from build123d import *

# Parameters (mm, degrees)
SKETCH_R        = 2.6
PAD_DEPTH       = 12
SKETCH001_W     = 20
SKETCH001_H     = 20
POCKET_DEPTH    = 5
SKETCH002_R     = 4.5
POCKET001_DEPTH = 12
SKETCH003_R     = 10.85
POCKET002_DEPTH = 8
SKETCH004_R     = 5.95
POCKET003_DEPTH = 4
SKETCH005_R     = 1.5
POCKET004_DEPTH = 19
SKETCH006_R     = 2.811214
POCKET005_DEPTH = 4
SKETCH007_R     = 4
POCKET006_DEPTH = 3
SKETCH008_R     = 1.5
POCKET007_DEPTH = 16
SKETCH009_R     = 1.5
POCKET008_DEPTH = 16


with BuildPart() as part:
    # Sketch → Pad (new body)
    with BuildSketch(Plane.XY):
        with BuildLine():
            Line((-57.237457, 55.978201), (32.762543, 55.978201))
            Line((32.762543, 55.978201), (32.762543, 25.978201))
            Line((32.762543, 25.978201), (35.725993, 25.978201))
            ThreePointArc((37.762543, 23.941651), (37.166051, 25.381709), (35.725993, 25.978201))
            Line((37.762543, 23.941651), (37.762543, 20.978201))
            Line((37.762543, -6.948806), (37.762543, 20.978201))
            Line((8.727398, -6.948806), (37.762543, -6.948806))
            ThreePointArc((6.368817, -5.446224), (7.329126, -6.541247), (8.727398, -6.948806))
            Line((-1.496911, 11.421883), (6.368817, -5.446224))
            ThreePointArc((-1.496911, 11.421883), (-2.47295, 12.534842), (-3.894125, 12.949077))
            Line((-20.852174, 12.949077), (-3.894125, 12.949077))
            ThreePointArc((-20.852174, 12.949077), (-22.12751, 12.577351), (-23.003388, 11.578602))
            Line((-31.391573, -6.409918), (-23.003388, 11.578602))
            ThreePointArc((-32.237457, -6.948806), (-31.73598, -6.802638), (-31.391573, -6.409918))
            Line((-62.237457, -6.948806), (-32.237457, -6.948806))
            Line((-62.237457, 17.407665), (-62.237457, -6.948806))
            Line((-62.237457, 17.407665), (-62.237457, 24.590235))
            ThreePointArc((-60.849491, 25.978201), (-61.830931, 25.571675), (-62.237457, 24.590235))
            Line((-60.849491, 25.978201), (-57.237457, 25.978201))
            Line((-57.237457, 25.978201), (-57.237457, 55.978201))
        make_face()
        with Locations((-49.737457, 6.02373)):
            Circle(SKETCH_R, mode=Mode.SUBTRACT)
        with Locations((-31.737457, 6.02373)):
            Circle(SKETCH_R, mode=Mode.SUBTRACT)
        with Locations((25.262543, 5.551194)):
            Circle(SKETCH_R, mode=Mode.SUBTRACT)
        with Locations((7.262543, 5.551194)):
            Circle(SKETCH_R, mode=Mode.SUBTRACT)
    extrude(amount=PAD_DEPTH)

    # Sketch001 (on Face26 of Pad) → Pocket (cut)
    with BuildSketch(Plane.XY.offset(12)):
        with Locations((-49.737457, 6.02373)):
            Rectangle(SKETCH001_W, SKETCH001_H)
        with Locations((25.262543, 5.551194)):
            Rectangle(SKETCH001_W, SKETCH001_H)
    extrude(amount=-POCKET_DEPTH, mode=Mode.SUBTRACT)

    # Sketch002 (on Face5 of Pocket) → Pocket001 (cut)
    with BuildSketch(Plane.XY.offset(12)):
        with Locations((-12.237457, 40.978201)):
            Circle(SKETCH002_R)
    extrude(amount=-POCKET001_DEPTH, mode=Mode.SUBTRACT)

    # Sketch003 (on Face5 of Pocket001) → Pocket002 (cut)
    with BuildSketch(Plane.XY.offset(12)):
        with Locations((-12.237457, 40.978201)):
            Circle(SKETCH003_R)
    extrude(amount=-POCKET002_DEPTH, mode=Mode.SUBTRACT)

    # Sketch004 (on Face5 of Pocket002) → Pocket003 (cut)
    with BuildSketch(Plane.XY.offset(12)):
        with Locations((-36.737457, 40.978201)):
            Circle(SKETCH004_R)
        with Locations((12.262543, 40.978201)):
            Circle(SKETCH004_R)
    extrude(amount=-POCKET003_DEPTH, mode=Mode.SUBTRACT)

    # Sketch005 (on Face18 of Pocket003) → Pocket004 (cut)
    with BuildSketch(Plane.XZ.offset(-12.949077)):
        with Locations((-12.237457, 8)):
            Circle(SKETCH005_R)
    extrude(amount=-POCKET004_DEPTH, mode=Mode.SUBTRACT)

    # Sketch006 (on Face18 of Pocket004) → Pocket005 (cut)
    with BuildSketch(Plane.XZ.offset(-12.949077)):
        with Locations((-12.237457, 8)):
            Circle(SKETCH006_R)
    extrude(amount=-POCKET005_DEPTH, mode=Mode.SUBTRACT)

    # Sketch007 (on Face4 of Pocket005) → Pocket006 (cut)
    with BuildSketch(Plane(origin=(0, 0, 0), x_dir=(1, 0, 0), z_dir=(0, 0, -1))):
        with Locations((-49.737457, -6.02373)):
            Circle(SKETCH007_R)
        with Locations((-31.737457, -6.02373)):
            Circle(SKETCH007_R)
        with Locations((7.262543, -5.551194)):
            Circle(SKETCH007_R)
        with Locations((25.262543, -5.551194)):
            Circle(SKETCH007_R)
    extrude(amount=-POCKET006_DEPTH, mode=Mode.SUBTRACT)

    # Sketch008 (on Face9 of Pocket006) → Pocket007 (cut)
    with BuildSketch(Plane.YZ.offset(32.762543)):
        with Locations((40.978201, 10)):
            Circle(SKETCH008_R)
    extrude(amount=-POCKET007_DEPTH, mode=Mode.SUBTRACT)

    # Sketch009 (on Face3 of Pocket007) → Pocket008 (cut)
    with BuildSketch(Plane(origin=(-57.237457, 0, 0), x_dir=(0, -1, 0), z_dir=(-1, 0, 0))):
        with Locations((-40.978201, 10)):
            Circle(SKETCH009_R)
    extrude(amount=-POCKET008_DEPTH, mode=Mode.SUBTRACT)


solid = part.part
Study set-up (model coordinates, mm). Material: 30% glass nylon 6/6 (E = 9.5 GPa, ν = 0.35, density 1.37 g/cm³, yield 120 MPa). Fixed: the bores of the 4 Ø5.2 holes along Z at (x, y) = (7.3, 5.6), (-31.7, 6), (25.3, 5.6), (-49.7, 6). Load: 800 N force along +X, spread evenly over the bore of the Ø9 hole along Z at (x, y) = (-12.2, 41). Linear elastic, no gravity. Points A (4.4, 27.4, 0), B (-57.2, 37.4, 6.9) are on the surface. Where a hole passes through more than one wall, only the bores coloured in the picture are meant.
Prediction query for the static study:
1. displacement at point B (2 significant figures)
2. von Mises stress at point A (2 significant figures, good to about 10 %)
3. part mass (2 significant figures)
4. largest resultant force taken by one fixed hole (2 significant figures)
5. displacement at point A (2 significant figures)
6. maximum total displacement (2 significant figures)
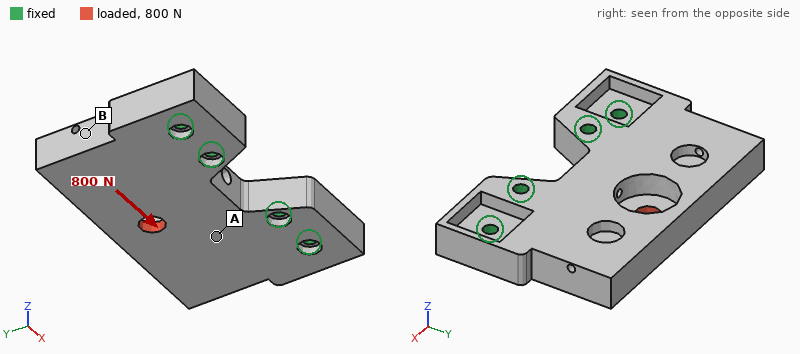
22 µm
2.9 MPa
76 g
350 N
12 µm
34 µm
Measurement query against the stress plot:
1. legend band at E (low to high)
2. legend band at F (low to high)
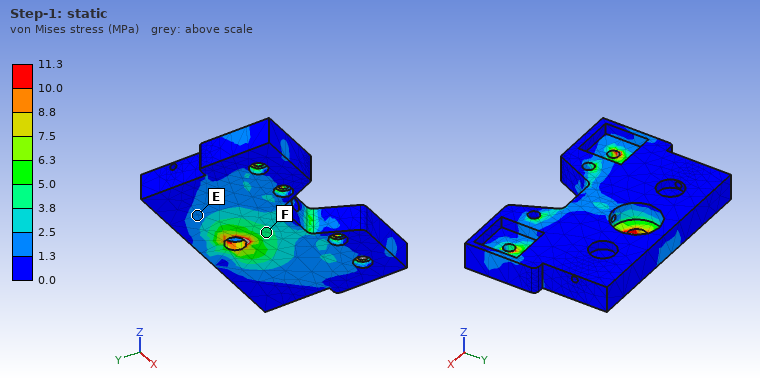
1.3 to 2.5 MPa
3.8 to 5.0 MPa
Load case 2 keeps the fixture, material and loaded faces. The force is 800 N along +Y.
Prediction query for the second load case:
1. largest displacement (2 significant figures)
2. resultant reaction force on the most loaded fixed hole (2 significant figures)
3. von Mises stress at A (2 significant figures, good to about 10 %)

65 µm
280 N
3.0 MPa
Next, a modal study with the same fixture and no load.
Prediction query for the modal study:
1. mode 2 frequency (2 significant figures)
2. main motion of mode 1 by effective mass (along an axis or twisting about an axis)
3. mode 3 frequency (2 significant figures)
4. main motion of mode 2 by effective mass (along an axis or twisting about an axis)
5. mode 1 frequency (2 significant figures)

2200 Hz
along Z
4800 Hz
twisting about Y
1400 Hz
